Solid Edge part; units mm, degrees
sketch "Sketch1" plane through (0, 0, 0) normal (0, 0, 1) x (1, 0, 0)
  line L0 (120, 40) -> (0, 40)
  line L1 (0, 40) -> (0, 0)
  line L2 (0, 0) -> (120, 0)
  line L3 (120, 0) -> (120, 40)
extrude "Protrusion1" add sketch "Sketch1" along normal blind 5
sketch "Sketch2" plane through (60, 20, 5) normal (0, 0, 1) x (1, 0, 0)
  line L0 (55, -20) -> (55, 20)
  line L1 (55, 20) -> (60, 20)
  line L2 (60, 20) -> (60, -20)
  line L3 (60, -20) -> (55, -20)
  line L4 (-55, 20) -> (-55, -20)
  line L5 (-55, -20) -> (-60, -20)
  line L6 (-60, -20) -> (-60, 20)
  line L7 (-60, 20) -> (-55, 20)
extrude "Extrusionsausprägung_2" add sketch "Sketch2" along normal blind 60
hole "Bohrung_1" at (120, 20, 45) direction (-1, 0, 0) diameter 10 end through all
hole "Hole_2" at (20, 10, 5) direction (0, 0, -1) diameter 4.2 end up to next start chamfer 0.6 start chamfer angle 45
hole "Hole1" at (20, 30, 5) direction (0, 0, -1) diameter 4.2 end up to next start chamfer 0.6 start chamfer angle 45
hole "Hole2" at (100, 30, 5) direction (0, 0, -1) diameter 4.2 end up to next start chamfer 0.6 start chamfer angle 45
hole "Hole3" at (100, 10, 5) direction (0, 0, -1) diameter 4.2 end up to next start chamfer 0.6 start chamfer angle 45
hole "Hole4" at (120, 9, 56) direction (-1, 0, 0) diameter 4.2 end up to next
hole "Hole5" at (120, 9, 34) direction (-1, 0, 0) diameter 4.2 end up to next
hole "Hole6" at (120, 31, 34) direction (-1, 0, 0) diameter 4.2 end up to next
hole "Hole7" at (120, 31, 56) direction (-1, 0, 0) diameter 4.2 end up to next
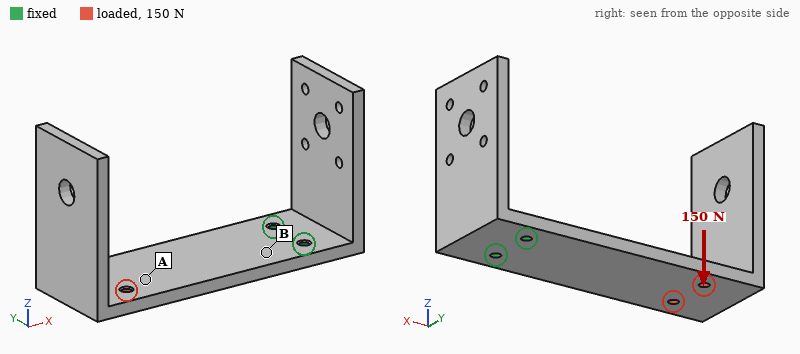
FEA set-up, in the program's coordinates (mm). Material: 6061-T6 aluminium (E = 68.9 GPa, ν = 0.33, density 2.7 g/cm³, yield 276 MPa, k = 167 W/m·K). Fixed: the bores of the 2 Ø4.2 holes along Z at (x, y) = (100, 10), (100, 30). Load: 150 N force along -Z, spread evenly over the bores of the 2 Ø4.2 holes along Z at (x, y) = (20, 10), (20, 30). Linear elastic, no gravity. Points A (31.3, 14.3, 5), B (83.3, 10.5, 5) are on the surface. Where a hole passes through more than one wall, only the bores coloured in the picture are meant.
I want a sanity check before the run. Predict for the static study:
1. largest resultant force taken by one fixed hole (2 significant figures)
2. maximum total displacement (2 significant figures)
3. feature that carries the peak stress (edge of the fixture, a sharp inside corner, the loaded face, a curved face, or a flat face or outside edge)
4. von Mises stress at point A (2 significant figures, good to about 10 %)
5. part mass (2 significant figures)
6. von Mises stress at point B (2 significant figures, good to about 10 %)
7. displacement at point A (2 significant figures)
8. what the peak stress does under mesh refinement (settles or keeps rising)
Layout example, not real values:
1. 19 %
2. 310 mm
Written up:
1. 76 N
2. 1.6 mm
3. edge of the fixture
4. 11 MPa
5. 130 g
6. 53 MPa
7. 0.70 mm
8. keeps rising
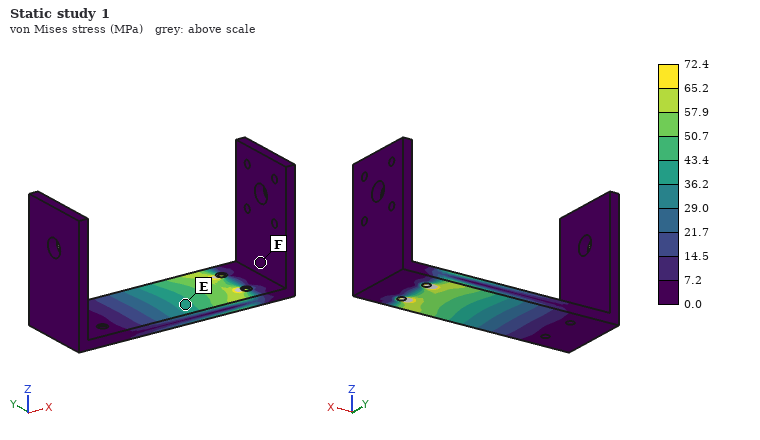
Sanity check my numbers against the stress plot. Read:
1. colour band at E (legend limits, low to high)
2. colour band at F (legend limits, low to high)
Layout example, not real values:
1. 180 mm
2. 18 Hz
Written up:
1. 36.2 to 43.4 MPa
2. 0.0 to 7.2 MPa
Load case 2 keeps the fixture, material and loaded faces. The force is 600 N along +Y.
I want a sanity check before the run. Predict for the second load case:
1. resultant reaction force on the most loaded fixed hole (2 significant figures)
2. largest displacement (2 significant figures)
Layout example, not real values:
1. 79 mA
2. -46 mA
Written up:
1. 2.2 kN
2. 0.11 mm
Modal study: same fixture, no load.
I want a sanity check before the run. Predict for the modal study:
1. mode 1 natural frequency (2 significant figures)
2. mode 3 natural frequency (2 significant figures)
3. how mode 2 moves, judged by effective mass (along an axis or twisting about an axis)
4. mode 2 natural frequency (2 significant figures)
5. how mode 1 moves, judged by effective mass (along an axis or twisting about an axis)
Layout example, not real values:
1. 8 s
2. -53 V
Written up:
1. 210 Hz
2. 710 Hz
3. along Y
4. 480 Hz
5. along Z
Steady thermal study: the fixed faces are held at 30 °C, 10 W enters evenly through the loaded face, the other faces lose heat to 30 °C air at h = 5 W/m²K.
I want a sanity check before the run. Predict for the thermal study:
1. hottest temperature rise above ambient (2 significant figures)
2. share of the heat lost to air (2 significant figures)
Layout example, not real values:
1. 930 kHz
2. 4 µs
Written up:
1. 23 K
2. 12 %
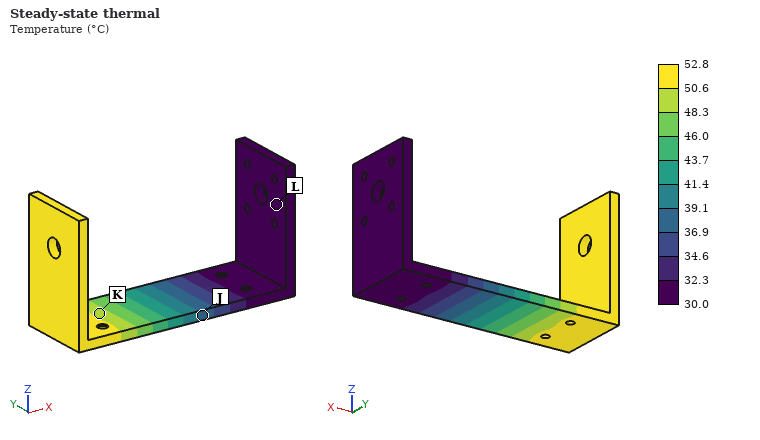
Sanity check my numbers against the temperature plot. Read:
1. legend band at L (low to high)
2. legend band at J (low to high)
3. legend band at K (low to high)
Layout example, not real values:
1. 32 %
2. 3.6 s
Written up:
1. 30.0 to 32.3 °C
2. 36.9 to 39.1 °C
3. 48.3 to 50.6 °C
